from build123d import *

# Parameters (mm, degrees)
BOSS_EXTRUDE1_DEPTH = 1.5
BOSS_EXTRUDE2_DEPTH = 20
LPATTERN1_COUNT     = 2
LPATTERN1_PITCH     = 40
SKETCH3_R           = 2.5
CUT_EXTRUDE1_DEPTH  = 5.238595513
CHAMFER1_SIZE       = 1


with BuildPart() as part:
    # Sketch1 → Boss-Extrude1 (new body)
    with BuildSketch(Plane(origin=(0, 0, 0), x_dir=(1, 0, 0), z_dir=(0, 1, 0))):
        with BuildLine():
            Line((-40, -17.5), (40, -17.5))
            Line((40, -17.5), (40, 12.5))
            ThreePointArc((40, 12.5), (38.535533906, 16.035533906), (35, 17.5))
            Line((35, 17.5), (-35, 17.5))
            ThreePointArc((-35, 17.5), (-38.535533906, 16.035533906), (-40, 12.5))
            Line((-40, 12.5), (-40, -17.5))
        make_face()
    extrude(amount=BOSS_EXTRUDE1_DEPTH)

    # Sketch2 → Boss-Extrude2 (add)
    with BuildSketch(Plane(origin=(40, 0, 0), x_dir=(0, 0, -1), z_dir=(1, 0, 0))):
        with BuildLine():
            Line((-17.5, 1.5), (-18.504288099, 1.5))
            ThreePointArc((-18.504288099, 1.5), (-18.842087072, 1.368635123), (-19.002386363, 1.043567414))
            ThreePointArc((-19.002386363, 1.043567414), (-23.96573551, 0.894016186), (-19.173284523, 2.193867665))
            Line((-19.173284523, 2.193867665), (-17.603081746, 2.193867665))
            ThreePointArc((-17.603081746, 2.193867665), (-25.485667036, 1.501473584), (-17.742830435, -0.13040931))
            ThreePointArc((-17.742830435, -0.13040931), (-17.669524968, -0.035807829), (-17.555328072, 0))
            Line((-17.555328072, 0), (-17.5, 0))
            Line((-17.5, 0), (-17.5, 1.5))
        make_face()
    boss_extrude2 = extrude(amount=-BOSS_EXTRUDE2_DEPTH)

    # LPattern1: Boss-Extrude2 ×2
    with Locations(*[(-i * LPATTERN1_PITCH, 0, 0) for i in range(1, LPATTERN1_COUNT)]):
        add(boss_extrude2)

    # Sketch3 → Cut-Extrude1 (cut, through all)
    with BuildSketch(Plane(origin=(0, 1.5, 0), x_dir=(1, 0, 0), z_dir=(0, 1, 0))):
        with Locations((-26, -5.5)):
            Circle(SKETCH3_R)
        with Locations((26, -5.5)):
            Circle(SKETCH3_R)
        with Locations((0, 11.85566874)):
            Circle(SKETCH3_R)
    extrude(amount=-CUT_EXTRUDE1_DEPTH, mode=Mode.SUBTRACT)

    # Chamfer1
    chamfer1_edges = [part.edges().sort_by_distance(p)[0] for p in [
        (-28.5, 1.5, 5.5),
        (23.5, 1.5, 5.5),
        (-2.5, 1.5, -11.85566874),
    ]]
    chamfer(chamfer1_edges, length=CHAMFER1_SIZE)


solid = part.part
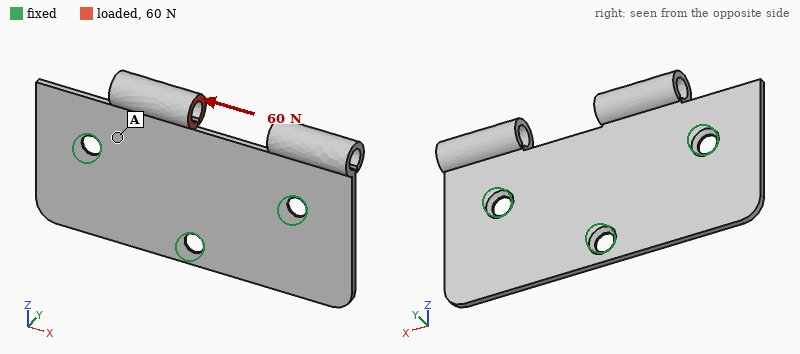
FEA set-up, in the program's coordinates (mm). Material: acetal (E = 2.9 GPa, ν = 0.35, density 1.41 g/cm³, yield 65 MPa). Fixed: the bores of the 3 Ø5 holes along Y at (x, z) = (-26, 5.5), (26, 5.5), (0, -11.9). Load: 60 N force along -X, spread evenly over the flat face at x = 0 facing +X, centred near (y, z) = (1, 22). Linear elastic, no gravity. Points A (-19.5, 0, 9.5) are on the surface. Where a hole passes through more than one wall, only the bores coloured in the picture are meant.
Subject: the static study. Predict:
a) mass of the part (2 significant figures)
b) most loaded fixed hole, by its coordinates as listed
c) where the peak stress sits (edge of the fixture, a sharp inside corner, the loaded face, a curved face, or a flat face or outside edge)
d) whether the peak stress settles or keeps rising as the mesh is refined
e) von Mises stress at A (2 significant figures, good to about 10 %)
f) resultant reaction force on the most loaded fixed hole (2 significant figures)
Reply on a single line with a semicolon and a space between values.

7.4 g; (-26, 5.5); a sharp inside corner; keeps rising; 3.0 MPa; 43 N
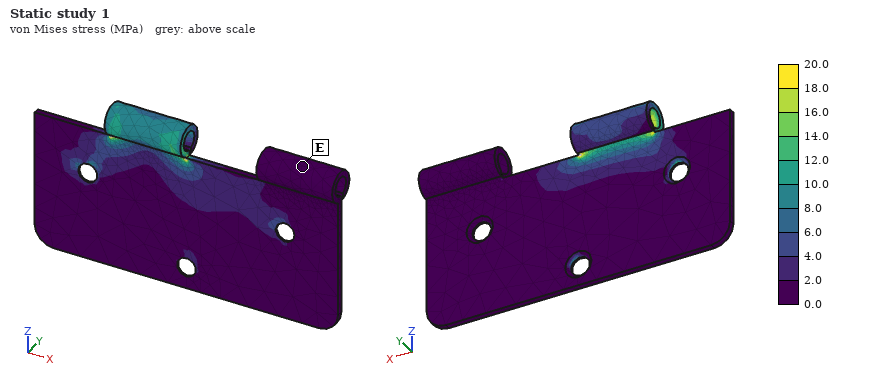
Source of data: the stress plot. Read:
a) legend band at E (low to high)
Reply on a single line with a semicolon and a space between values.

0.0 to 2.0 MPa
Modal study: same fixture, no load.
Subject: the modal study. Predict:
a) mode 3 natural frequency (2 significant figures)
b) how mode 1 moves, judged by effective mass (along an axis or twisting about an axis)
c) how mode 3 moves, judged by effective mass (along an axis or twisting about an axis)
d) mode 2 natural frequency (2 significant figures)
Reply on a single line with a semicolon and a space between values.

780 Hz; along Y; twisting about Z; 550 Hz
